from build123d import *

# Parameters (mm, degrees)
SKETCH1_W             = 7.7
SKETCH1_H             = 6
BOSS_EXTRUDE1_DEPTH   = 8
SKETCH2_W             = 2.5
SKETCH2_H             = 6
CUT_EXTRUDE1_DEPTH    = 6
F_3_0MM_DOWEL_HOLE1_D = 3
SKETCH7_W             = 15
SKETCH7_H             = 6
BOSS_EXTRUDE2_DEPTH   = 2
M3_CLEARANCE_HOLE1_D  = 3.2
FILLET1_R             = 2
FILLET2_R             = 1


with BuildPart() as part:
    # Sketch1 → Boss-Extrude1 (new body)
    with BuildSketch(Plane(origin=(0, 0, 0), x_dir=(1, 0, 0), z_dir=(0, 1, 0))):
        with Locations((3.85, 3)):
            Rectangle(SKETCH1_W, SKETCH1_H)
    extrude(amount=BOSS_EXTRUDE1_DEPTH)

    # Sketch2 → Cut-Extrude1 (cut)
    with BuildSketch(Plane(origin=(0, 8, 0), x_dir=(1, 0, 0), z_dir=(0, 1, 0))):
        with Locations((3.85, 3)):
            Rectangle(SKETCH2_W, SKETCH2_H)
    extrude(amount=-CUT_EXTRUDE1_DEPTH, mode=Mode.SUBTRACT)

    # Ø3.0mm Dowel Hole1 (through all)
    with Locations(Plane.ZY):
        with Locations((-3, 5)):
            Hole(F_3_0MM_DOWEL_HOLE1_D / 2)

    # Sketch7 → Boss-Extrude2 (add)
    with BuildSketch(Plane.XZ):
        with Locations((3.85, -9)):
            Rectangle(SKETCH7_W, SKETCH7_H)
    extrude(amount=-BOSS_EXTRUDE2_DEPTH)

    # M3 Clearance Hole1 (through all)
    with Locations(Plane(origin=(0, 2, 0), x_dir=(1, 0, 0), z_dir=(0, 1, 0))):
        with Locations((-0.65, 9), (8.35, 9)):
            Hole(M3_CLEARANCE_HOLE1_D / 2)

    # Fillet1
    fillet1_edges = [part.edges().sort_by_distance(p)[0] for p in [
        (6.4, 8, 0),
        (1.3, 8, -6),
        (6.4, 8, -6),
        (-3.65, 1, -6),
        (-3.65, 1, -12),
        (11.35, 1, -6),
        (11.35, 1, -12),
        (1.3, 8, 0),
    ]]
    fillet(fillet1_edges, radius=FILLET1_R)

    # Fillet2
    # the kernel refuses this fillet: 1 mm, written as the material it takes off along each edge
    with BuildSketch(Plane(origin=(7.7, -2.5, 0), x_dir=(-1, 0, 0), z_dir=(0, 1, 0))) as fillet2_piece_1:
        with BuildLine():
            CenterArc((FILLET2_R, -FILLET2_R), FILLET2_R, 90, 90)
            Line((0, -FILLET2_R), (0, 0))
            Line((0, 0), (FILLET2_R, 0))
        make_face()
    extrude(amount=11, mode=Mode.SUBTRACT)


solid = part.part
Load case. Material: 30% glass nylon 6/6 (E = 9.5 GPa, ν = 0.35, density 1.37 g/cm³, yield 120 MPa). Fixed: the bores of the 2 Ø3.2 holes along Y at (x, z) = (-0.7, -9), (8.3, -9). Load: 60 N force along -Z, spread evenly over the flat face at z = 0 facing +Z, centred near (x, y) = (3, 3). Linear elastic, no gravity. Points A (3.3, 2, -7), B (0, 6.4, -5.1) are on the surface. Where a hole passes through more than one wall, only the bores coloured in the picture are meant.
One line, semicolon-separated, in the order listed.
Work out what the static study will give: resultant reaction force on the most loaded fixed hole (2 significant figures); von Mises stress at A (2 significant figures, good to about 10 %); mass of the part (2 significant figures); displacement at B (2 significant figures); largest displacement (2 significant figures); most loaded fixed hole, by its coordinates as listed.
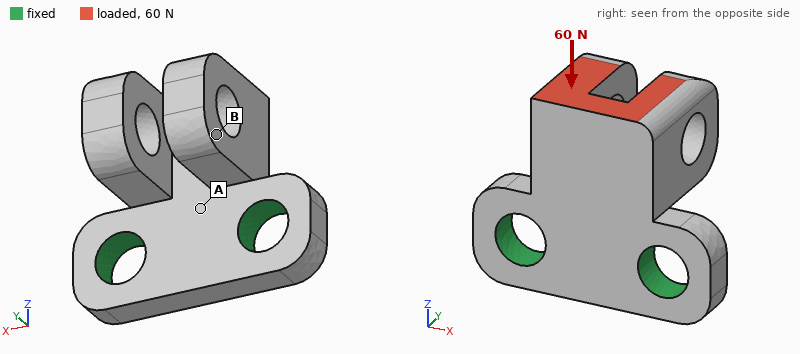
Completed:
37 N; 12 MPa; 0.51 g; 40 µm; 60 µm; (-0.7, -9)
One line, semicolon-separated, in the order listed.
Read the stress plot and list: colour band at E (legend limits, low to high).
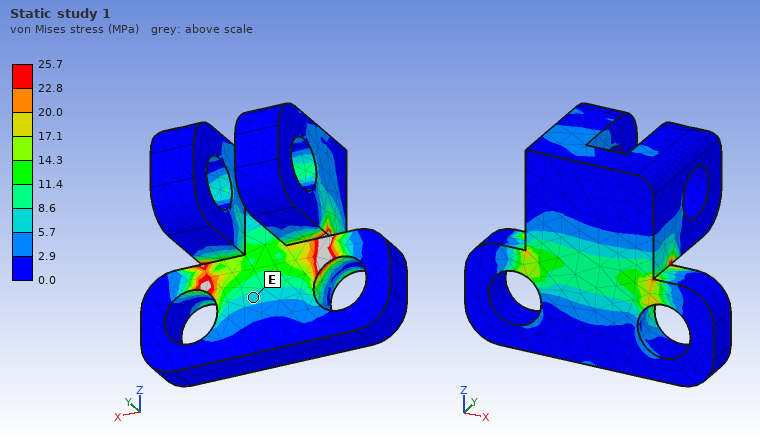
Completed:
5.7 to 8.6 MPa
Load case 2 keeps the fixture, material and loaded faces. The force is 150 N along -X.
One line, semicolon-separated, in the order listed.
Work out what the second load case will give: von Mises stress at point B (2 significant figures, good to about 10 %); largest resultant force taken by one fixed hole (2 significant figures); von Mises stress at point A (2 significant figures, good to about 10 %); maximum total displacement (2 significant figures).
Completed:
6.7 MPa; 170 N; 13 MPa; 0.12 mm
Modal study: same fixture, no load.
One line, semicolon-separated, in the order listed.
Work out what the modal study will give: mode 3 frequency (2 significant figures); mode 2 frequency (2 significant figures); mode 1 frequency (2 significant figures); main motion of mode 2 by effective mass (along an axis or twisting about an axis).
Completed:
16 kHz; 12 kHz; 6700 Hz; along X
